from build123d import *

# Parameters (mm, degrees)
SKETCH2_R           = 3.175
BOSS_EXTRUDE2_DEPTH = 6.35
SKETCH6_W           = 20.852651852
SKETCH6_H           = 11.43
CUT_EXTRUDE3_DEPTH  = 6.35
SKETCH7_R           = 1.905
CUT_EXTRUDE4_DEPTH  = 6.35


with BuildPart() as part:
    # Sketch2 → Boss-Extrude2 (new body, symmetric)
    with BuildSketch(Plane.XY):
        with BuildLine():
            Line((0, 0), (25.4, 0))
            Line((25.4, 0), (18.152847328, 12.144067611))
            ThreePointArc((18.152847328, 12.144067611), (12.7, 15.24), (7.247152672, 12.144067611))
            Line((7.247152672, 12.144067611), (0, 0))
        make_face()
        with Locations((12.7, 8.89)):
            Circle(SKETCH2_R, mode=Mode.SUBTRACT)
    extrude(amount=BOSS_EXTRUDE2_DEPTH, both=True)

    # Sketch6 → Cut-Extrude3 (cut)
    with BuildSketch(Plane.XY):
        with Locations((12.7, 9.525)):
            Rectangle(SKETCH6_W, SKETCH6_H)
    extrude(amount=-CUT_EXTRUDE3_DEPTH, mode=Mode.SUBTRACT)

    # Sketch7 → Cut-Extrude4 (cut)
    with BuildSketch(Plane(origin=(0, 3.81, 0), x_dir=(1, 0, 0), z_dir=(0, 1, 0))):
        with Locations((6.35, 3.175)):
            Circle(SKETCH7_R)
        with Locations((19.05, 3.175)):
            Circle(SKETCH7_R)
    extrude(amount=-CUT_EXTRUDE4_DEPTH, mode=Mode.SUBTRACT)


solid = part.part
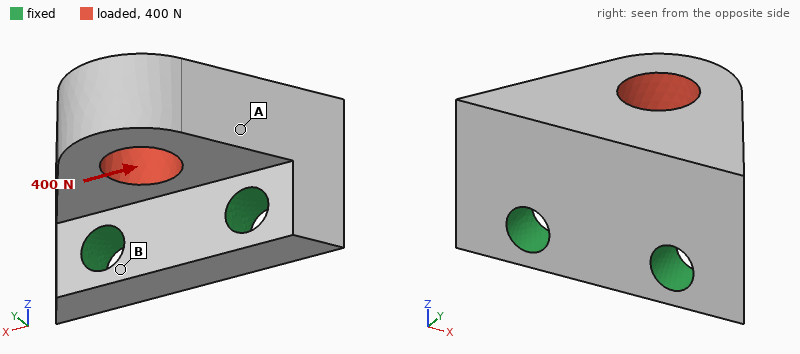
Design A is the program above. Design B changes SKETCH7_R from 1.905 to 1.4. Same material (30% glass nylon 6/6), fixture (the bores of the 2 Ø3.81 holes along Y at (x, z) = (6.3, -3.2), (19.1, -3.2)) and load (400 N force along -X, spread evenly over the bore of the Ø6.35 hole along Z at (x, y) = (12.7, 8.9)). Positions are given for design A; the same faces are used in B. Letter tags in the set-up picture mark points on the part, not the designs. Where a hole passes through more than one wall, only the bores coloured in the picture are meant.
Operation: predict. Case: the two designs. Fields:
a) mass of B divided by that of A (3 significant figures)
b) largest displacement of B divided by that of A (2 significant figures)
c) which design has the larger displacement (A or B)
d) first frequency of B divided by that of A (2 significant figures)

1.02
1.2
B
0.90
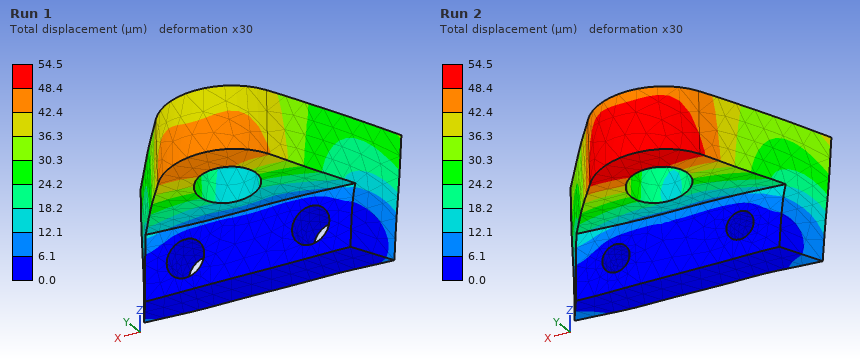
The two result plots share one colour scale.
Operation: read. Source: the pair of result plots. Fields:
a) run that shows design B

Run 2
